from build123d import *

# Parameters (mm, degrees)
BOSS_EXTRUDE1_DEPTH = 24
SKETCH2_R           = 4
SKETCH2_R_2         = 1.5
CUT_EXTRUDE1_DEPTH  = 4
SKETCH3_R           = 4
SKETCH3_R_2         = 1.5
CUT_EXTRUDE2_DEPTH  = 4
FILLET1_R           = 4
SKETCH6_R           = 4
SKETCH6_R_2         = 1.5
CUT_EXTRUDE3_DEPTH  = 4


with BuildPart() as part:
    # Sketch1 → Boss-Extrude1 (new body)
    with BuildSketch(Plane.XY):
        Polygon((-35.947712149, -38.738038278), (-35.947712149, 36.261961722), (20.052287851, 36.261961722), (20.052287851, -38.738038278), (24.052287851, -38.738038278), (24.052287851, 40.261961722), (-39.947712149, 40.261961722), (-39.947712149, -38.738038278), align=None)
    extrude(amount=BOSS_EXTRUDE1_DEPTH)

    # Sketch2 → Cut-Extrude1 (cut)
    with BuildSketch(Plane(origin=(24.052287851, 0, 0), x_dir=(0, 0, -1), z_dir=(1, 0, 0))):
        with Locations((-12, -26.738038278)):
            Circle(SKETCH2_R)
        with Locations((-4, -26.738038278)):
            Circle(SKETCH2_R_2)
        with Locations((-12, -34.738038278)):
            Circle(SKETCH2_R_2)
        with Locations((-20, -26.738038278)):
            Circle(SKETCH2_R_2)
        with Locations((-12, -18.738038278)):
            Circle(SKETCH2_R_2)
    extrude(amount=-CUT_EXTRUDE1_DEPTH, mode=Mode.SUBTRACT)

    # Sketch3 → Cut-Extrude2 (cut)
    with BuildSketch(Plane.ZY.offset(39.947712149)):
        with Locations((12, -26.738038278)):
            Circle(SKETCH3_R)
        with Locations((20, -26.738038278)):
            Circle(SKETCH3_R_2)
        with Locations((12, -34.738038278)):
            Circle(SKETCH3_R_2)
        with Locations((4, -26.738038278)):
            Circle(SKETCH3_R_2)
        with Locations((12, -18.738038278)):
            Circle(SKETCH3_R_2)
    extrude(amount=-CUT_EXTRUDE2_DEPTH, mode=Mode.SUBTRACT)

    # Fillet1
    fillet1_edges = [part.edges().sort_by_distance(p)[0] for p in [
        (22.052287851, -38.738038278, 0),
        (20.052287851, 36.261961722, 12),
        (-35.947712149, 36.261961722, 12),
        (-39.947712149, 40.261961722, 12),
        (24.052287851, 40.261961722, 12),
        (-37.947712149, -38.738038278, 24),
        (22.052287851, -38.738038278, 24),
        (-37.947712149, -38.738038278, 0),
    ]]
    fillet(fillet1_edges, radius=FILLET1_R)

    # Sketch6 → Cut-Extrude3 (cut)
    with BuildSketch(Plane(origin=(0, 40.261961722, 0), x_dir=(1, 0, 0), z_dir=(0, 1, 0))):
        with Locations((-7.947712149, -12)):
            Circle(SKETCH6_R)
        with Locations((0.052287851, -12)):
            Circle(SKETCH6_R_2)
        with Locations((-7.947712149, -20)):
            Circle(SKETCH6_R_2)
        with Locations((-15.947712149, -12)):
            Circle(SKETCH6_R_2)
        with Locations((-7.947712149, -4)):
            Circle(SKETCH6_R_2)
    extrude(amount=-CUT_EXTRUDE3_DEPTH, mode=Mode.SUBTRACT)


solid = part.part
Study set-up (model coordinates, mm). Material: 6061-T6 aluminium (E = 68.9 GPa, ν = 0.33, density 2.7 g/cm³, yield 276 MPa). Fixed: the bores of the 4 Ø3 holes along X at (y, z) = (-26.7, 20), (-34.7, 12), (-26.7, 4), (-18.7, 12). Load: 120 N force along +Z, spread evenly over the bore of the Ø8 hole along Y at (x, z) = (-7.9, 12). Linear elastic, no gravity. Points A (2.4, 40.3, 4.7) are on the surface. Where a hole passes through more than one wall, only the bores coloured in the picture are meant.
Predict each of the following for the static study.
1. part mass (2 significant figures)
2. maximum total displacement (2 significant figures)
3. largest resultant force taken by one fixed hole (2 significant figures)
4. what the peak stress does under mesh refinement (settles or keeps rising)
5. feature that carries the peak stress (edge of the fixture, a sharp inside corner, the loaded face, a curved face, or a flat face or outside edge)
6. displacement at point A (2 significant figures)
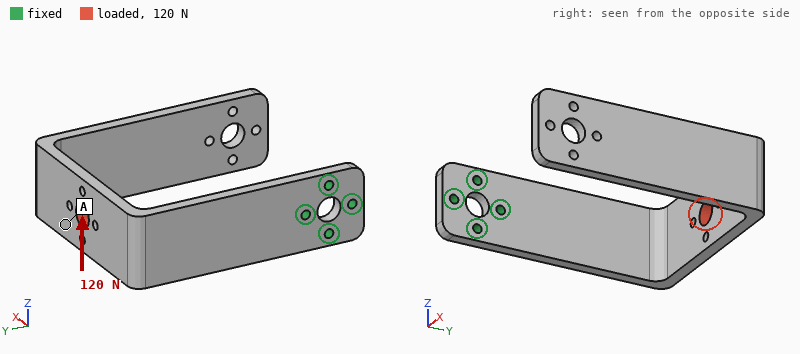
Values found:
53 g
1.0 mm
340 N
keeps rising
edge of the fixture
0.68 mm
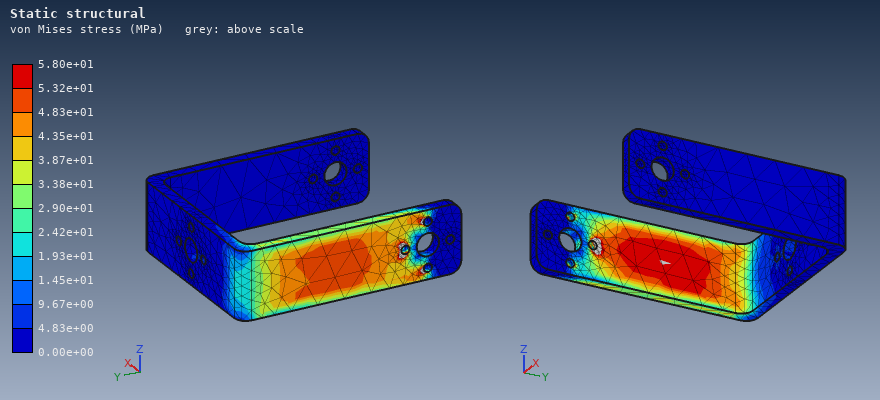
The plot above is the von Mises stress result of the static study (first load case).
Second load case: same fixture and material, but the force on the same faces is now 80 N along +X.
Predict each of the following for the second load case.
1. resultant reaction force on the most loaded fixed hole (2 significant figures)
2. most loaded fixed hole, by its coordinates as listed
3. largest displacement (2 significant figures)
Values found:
350 N
(-18.7, 12)
1.1 mm
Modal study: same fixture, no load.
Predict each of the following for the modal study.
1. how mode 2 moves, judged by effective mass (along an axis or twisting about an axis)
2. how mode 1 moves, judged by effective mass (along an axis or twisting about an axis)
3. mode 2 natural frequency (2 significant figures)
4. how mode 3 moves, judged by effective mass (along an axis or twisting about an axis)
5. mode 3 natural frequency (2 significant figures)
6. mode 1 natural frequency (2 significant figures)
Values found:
along Z
along Y
220 Hz
along X
330 Hz
160 Hz
